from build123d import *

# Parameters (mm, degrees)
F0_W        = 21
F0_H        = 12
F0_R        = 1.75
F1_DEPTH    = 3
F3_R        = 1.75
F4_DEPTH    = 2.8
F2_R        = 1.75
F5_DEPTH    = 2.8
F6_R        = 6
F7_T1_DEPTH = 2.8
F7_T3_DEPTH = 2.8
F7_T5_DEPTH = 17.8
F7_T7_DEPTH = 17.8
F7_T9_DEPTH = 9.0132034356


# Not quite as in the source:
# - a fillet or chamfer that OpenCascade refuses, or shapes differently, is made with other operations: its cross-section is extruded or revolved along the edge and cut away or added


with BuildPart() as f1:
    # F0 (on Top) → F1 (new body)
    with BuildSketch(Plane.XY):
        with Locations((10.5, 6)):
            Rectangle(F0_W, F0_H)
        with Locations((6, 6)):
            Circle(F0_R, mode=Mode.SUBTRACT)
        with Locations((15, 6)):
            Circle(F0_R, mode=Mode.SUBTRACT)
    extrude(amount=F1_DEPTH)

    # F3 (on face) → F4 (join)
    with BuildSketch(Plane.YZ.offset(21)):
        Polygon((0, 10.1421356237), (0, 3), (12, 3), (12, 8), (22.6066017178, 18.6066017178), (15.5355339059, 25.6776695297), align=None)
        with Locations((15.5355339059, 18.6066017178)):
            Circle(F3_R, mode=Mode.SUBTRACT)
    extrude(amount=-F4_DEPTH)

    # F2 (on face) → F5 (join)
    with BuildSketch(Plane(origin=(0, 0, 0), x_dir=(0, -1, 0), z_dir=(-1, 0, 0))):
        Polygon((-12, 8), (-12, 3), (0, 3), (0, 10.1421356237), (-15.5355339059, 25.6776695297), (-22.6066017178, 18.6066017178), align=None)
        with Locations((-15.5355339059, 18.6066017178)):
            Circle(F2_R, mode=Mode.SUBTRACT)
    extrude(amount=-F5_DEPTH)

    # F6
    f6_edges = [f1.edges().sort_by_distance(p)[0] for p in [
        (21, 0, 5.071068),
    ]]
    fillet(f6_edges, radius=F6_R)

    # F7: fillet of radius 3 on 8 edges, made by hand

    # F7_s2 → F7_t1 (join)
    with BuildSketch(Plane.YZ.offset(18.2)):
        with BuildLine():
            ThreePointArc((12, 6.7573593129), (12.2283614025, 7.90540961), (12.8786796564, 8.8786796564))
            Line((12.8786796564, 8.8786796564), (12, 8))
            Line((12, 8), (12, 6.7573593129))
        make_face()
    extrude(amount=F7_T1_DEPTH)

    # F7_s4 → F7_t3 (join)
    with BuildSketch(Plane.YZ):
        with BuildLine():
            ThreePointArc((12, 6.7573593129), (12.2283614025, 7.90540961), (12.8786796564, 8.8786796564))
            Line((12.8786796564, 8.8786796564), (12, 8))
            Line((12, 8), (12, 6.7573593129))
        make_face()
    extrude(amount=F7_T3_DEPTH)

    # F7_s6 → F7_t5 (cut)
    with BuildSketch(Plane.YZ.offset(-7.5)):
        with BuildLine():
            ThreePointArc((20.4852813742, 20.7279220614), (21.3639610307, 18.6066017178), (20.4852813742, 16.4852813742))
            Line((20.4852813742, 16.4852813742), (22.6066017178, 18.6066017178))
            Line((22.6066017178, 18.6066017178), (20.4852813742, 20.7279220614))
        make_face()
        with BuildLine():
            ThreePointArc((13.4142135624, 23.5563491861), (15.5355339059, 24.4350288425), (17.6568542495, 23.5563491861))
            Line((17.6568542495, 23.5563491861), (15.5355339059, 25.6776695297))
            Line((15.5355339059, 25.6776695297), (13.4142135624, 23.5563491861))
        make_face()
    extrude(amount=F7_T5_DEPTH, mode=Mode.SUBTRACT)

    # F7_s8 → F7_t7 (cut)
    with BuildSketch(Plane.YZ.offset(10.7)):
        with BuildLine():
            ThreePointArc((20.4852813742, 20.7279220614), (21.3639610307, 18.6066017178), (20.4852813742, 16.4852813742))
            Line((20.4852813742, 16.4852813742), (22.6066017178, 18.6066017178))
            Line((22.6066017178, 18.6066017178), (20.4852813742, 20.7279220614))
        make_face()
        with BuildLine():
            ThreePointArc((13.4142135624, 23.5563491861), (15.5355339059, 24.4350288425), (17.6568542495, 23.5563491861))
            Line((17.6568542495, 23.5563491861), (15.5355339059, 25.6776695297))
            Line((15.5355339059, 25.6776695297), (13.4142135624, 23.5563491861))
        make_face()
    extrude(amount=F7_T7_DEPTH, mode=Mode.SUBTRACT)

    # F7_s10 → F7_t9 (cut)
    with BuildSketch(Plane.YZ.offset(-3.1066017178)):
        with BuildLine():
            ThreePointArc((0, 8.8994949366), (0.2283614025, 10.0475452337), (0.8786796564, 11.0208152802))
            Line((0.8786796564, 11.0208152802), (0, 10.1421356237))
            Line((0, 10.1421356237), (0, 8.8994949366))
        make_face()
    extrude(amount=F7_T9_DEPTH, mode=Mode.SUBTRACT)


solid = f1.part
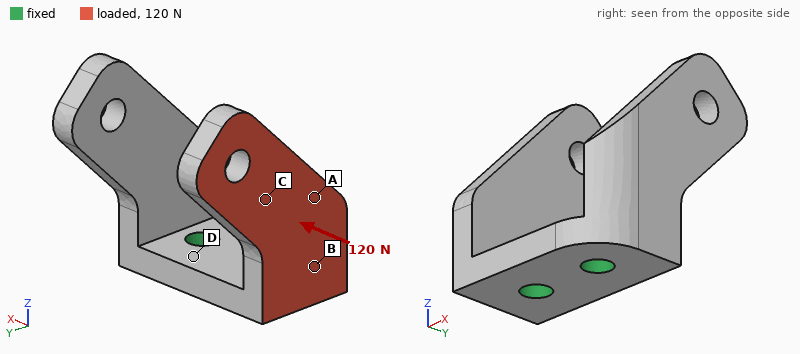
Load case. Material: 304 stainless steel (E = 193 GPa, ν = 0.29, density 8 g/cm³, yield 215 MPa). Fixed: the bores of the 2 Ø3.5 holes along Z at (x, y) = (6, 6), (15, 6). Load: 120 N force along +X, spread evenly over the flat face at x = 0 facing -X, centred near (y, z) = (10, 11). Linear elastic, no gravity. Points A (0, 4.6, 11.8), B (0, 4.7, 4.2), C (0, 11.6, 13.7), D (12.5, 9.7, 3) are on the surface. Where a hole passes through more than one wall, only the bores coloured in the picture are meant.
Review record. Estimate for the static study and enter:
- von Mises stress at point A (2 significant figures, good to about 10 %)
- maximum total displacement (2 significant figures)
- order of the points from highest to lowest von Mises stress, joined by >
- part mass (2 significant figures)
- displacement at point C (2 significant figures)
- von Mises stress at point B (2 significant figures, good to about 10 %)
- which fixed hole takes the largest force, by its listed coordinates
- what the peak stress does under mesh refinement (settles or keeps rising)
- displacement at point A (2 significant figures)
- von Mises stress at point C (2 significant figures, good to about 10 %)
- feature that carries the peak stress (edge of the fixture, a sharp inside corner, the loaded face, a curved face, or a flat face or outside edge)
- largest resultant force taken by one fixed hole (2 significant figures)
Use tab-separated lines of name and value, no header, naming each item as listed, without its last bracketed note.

von Mises stress at point A	30 MPa
maximum total displacement	60 µm
order of the points from highest to lowest von Mises stress, joined by >	B > A > C > D
part mass	16 g
displacement at point C	26 µm
von Mises stress at point B	55 MPa
which fixed hole takes the largest force, by its listed coordinates	(6, 6)
what the peak stress does under mesh refinement	keeps rising
displacement at point A	17 µm
von Mises stress at point C	18 MPa
feature that carries the peak stress	edge of the fixture
largest resultant force taken by one fixed hole	110 N
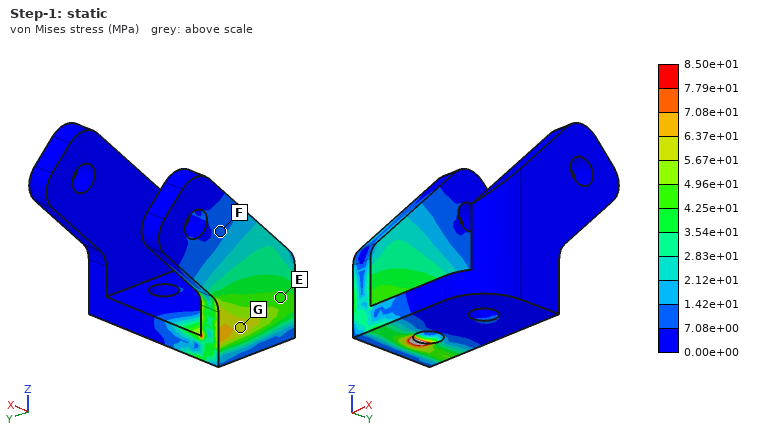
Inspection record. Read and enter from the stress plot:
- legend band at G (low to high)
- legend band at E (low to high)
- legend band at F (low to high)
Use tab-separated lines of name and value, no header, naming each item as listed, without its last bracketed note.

legend band at G	5.67e+01 to 6.37e+01 MPa
legend band at E	4.25e+01 to 4.96e+01 MPa
legend band at F	7.08e+00 to 1.42e+01 MPa
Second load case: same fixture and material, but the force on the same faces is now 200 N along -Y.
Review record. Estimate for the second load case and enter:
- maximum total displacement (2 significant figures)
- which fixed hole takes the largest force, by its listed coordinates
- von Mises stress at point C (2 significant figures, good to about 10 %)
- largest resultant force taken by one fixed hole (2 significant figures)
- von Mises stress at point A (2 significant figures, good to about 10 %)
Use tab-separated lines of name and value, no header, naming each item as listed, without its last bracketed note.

maximum total displacement	23 µm
which fixed hole takes the largest force, by its listed coordinates	(6, 6)
von Mises stress at point C	12 MPa
largest resultant force taken by one fixed hole	260 N
von Mises stress at point A	15 MPa
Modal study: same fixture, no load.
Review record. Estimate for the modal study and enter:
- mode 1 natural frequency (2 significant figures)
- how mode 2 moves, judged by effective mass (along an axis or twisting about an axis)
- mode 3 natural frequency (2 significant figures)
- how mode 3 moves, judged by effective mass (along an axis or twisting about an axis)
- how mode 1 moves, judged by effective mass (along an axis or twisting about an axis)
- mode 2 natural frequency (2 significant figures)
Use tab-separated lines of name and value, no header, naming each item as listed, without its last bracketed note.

mode 1 natural frequency	3400 Hz
how mode 2 moves, judged by effective mass	along X
mode 3 natural frequency	6700 Hz
how mode 3 moves, judged by effective mass	along Y
how mode 1 moves, judged by effective mass	along X
mode 2 natural frequency	3700 Hz
